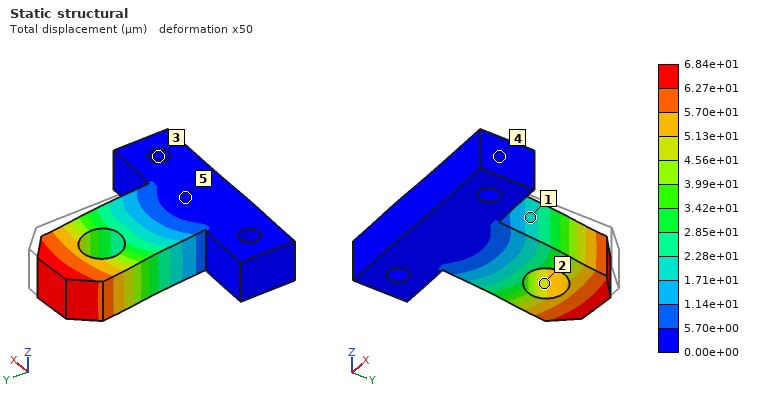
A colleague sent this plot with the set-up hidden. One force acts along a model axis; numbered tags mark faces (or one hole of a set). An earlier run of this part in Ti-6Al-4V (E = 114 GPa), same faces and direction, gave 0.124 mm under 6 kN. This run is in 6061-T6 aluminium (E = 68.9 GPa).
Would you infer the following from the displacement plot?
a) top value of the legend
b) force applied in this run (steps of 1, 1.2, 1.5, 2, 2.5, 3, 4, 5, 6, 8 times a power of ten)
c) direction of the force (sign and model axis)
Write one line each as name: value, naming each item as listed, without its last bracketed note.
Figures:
top value of the legend: 6.84e+01 µm
force applied in this run: 2 kN
direction of the force: -X
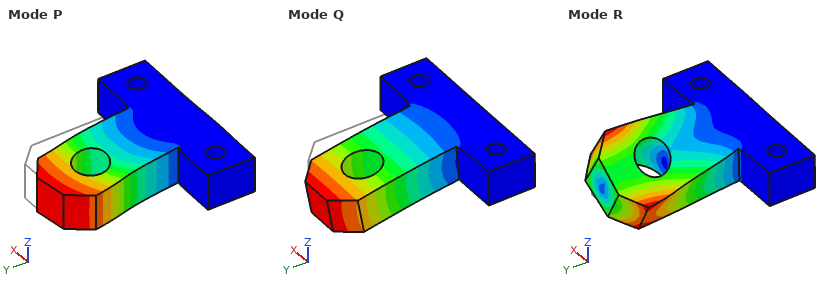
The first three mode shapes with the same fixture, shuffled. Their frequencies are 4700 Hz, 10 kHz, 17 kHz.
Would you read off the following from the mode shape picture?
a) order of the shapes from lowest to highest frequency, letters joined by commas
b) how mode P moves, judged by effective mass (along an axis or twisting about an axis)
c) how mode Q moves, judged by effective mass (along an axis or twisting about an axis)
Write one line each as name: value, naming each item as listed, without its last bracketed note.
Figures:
order of the shapes from lowest to highest frequency, letters joined by commas: Q, P, R
how mode P moves, judged by effective mass: along X
how mode Q moves, judged by effective mass: along Z
